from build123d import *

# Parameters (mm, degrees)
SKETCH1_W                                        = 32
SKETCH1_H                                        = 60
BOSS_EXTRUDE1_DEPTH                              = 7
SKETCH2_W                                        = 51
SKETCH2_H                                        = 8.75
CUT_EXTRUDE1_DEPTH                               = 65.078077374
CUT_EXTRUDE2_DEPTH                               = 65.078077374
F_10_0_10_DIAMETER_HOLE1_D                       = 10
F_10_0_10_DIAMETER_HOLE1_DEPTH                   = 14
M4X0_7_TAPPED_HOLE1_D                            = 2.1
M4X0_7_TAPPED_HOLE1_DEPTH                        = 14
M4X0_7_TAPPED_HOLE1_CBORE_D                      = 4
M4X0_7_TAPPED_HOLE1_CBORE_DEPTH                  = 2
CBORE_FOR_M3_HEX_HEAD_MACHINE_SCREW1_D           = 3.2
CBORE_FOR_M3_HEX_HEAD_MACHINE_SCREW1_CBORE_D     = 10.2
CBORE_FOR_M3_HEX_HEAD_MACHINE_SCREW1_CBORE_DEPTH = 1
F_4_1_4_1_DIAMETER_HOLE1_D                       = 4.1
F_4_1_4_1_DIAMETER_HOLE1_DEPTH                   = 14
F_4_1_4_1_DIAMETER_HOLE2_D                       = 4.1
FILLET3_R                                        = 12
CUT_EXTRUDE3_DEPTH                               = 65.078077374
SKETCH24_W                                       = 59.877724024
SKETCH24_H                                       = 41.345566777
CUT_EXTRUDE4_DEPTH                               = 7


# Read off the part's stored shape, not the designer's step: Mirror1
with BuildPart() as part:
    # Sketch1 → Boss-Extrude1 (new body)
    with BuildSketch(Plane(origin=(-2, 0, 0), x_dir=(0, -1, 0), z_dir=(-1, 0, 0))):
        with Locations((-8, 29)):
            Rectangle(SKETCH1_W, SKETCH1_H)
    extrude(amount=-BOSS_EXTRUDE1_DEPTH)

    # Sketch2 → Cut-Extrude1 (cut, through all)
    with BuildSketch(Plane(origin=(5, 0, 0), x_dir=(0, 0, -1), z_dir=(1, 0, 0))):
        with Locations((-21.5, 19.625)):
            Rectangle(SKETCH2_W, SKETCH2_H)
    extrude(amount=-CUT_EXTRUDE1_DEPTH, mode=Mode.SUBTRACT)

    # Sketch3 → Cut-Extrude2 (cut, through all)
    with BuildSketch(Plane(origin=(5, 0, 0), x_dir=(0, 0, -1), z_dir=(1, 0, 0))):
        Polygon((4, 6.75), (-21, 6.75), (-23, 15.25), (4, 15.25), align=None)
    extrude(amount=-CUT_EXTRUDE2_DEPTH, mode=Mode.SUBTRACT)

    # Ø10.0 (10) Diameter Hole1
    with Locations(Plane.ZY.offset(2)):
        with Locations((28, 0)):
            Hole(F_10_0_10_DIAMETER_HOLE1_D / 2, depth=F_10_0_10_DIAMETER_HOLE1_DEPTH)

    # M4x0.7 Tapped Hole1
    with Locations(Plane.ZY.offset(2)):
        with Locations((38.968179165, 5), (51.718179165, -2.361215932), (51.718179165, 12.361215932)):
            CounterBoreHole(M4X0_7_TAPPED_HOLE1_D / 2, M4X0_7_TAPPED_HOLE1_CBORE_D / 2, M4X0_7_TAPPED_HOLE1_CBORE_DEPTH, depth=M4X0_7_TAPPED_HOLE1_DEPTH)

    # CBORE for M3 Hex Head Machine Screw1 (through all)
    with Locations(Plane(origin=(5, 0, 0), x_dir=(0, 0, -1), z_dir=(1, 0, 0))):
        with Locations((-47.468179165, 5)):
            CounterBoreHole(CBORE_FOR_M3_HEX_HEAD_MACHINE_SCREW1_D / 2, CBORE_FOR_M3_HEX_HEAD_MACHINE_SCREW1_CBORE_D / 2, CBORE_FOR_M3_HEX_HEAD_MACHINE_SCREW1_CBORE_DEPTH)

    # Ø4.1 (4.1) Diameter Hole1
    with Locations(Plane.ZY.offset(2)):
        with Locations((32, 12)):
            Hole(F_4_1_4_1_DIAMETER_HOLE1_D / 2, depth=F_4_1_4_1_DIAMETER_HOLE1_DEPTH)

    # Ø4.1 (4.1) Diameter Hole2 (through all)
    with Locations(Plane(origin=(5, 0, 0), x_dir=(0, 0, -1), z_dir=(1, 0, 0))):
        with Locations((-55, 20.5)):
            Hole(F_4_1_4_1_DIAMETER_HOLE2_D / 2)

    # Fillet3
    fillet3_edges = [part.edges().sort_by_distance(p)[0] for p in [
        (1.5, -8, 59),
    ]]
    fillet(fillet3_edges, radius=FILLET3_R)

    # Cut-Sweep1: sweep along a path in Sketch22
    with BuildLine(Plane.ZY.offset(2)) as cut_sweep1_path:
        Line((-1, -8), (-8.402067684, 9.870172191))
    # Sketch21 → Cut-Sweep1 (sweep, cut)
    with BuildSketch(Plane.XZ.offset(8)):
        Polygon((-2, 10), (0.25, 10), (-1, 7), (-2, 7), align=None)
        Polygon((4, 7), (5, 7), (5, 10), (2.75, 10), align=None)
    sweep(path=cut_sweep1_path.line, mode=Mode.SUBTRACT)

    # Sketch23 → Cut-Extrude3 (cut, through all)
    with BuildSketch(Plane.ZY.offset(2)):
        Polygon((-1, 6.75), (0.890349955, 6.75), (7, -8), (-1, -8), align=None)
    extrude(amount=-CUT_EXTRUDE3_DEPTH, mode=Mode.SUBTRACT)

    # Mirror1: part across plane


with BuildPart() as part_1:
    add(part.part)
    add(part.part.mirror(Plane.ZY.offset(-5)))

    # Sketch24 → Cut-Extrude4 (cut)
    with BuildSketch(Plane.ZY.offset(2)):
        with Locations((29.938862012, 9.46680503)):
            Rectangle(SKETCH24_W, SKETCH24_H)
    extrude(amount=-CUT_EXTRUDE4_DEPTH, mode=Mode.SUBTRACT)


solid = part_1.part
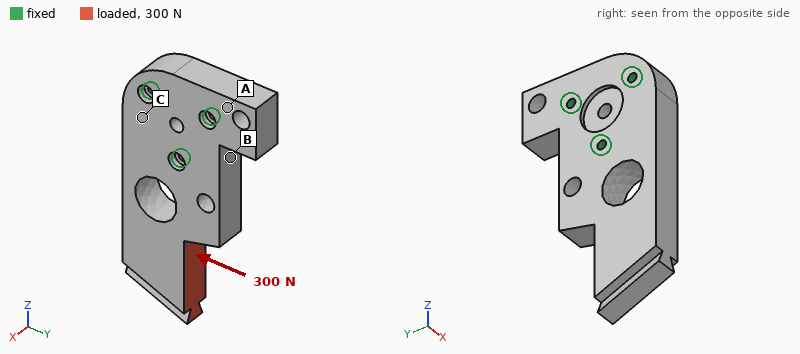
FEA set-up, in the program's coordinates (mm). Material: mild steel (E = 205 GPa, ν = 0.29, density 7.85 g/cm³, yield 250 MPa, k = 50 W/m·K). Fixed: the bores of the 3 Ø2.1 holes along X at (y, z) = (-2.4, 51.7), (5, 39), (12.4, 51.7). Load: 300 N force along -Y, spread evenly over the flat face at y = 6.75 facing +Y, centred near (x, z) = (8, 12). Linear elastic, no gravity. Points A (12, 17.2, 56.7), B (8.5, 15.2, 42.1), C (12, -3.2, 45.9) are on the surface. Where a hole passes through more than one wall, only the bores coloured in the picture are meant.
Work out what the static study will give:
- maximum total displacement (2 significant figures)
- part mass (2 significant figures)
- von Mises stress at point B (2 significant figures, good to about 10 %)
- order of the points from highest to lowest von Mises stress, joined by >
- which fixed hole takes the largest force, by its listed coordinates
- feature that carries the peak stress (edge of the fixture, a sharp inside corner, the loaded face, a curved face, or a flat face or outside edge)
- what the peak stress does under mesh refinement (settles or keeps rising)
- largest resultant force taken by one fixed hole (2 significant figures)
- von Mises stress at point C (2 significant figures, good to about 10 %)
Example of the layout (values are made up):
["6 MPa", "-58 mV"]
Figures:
["8.6 µm", "57 g", "14 MPa", "B > C > A", "(5, 39)", "edge of the fixture", "keeps rising", "530 N", "6.1 MPa"]
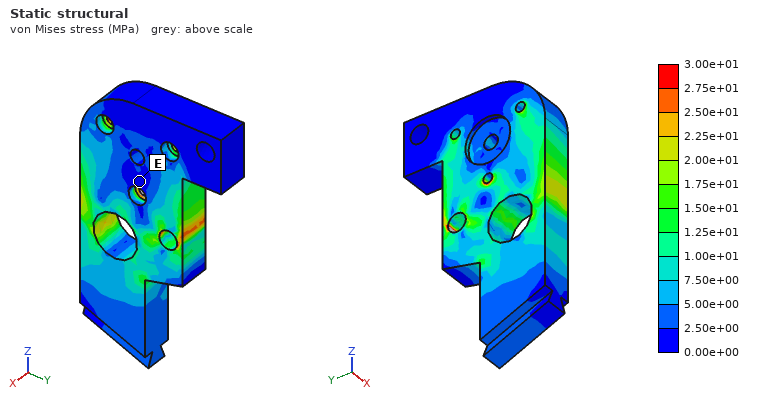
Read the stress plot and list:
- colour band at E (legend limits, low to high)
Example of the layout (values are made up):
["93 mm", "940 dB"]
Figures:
["0.00e+00 to 2.50e+00 MPa"]
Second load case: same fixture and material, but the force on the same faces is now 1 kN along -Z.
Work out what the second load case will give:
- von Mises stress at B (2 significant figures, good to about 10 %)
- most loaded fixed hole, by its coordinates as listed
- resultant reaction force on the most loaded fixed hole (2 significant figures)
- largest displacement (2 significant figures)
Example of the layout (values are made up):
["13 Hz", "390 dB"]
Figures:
["8.3 MPa", "(5, 39)", "620 N", "9.6 µm"]
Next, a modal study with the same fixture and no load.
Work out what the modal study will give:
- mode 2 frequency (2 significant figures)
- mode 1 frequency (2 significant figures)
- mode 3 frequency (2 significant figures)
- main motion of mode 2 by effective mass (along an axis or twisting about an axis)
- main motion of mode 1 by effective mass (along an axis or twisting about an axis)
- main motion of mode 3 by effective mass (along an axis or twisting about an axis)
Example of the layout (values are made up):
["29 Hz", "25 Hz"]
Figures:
["9500 Hz", "4000 Hz", "13 kHz", "along Y", "along X", "twisting about Z"]
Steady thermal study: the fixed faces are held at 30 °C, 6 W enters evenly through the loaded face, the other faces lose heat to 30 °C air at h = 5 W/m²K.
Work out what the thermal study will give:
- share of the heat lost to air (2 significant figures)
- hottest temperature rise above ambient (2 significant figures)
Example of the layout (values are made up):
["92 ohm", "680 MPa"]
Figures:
["3.8 %", "46 K"]
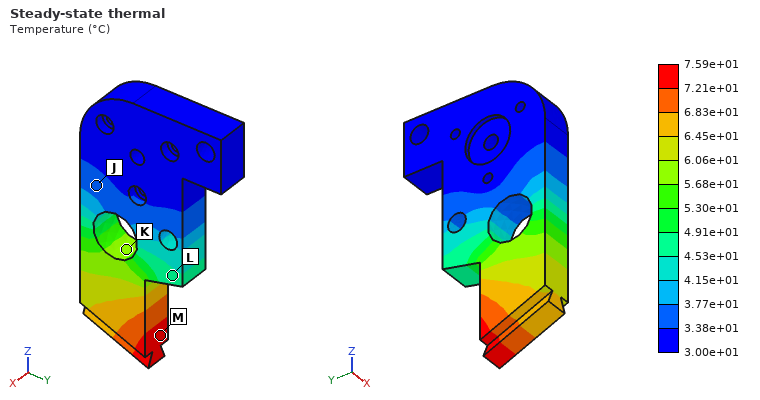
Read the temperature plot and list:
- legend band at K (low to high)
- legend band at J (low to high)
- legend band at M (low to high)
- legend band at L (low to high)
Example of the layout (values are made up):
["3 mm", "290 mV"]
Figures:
["5.68e+01 to 6.06e+01 °C", "3.38e+01 to 3.77e+01 °C", "7.21e+01 to 7.59e+01 °C", "4.53e+01 to 4.91e+01 °C"]
